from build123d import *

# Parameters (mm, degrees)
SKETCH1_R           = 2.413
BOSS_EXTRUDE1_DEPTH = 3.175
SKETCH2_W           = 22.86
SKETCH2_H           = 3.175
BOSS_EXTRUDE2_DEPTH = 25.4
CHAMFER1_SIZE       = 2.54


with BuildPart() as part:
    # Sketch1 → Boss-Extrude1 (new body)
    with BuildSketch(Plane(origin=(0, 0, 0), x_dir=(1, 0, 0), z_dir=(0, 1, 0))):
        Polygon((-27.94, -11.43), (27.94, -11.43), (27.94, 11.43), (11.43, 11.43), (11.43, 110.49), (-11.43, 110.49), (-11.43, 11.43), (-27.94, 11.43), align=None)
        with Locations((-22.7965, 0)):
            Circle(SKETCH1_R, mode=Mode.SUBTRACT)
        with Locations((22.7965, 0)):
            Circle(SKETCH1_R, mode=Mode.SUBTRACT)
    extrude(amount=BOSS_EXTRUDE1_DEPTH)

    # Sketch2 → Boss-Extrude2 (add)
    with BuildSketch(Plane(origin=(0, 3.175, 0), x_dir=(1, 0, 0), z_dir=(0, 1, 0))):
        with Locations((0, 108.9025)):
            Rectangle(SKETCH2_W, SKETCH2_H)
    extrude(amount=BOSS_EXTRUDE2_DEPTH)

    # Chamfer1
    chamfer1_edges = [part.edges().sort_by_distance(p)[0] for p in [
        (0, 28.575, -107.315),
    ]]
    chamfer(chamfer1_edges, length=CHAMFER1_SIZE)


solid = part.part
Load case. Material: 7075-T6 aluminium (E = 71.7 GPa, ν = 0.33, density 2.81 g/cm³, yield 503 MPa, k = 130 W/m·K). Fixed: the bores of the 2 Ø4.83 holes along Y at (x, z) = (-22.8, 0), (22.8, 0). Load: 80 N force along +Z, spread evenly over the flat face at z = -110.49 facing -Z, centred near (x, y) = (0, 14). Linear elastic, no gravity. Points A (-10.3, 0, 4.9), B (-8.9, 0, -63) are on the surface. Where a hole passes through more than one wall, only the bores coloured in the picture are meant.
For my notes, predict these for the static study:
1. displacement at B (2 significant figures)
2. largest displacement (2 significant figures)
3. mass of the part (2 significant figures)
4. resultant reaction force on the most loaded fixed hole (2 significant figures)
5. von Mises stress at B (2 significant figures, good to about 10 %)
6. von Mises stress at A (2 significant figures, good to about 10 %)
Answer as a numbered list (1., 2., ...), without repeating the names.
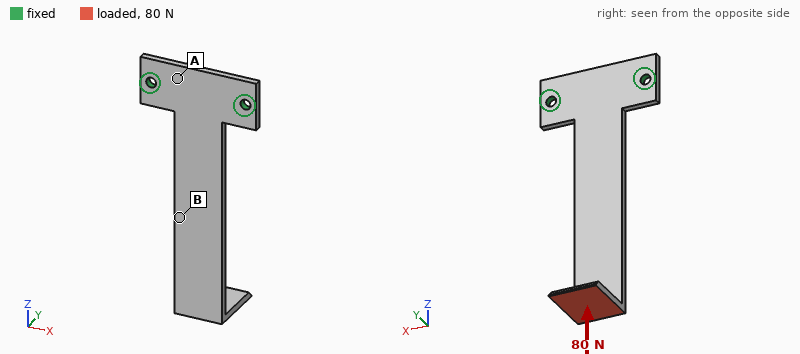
1. 0.45 mm
2. 1.6 mm
3. 36 g
4. 41 N
5. 25 MPa
6. 5.2 MPa
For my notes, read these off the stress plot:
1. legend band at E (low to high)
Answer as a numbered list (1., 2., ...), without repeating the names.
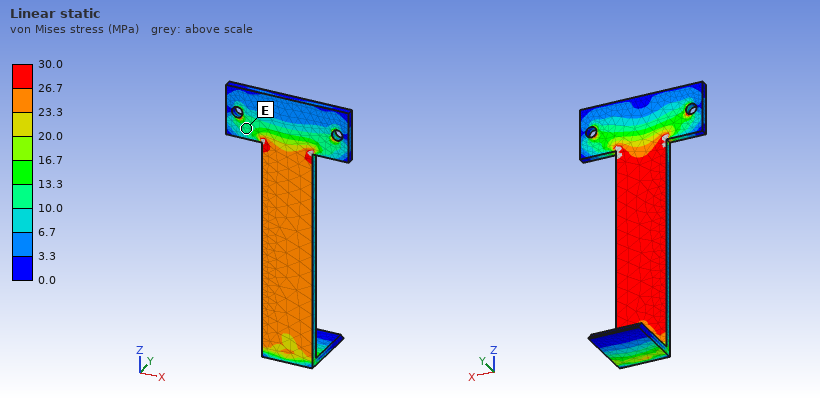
1. 10.0 to 13.3 MPa
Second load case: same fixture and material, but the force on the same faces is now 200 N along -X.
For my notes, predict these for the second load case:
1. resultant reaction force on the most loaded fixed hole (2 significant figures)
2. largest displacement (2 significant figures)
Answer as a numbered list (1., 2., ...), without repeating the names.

1. 530 N
2. 1.5 mm
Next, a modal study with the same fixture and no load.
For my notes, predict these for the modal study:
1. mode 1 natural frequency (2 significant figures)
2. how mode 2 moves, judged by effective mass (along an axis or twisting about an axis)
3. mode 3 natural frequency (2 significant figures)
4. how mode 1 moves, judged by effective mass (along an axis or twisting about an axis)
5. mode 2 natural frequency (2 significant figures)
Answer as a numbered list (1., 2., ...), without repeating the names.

1. 160 Hz
2. along X
3. 960 Hz
4. along Y
5. 840 Hz
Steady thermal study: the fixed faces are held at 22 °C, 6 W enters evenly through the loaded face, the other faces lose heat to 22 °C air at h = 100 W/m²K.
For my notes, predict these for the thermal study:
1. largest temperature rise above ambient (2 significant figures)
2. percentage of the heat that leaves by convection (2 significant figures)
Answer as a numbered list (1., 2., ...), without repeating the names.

1. 24 K
2. 90 %
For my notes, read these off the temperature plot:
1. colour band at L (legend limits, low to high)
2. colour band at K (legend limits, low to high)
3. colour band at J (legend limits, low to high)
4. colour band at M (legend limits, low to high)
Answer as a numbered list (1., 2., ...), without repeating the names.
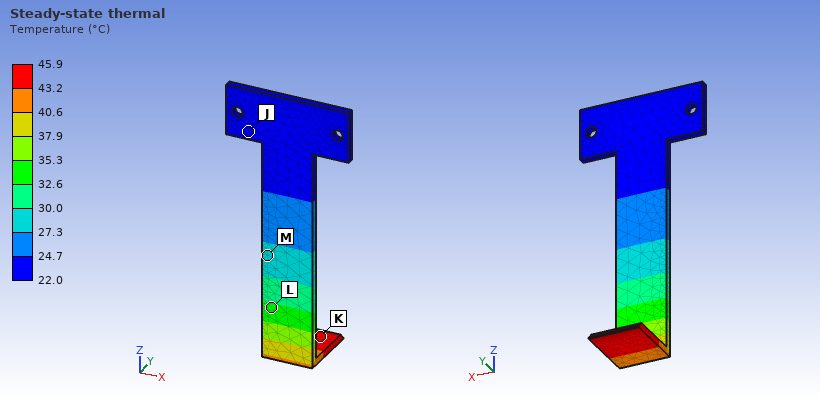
1. 32.6 to 35.3 °C
2. 43.2 to 45.9 °C
3. 22.0 to 24.7 °C
4. 27.3 to 30.0 °C
